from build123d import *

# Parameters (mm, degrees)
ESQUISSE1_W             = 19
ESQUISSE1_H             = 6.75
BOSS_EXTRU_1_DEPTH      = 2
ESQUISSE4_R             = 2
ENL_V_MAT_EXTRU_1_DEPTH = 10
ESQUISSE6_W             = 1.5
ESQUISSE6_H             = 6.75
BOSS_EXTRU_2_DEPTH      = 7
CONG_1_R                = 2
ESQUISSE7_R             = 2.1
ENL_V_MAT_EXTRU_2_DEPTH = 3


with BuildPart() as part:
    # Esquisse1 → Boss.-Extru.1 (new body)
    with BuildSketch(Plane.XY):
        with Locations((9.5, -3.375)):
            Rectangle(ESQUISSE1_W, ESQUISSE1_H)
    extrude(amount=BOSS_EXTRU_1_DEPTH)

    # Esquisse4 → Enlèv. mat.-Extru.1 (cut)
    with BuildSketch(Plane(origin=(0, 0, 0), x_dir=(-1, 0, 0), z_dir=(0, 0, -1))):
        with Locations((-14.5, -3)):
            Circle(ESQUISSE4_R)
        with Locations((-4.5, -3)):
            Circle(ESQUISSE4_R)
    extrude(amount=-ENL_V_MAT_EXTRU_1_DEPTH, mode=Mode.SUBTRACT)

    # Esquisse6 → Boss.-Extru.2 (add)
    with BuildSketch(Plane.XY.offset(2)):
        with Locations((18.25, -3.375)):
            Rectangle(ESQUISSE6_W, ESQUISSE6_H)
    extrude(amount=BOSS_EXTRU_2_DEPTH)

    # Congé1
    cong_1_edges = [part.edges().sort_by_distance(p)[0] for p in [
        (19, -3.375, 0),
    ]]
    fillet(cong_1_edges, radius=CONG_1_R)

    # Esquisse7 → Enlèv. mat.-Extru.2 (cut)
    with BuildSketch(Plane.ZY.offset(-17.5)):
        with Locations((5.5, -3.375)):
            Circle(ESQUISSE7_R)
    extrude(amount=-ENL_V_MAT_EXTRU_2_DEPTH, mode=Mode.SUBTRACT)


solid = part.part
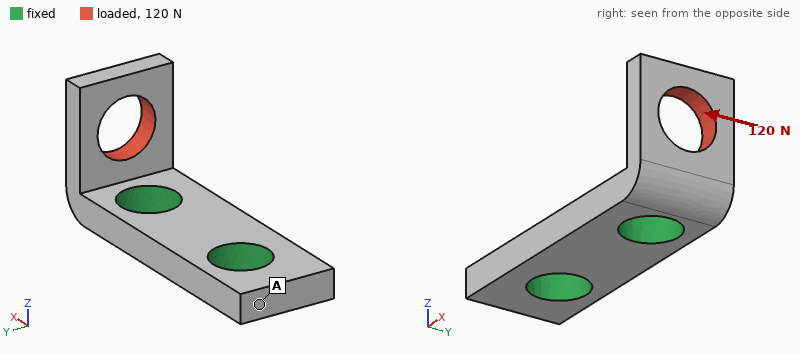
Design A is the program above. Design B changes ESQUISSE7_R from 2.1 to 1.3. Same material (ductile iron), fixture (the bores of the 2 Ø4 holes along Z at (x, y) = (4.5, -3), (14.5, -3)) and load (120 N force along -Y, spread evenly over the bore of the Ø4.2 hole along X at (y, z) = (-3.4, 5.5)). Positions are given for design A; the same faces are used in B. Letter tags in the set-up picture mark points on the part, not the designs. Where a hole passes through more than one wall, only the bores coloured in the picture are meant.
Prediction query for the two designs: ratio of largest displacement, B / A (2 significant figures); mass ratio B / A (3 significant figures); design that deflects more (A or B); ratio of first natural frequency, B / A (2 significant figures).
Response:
0.75
1.05
A
1.0
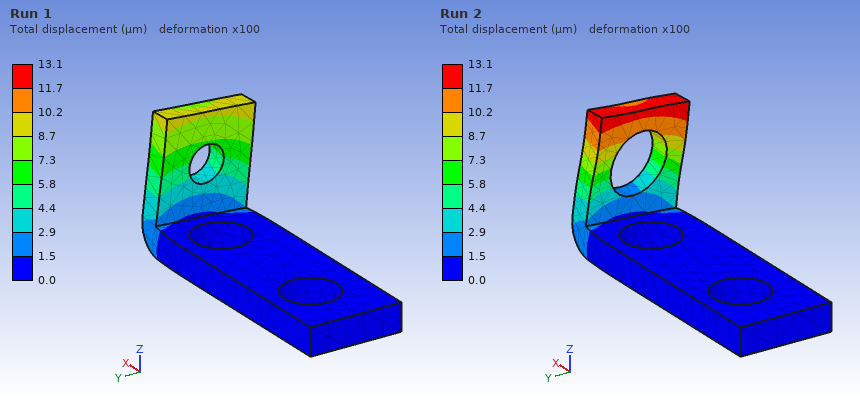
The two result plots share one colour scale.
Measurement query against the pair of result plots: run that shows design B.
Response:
Run 1
